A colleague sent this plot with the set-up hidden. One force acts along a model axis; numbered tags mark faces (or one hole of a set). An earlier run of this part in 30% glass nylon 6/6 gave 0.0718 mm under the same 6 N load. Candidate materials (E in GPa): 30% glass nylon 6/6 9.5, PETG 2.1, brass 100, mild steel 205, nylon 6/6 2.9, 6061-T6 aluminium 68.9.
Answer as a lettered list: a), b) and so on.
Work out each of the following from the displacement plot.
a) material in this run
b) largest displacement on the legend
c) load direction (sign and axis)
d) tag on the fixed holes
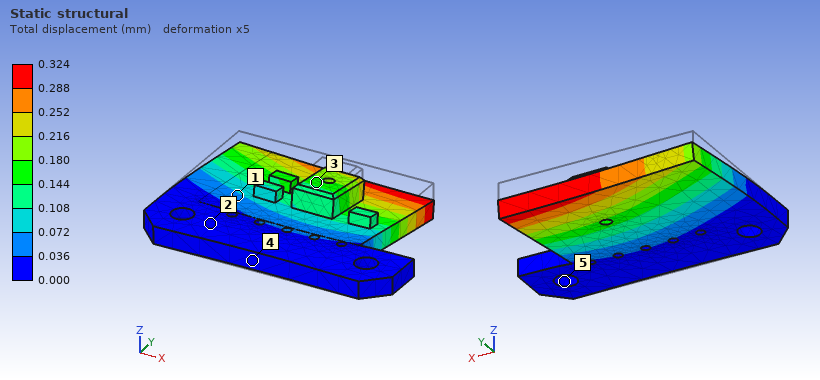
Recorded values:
a) PETG
b) 0.324 mm
c) -Z
d) 5
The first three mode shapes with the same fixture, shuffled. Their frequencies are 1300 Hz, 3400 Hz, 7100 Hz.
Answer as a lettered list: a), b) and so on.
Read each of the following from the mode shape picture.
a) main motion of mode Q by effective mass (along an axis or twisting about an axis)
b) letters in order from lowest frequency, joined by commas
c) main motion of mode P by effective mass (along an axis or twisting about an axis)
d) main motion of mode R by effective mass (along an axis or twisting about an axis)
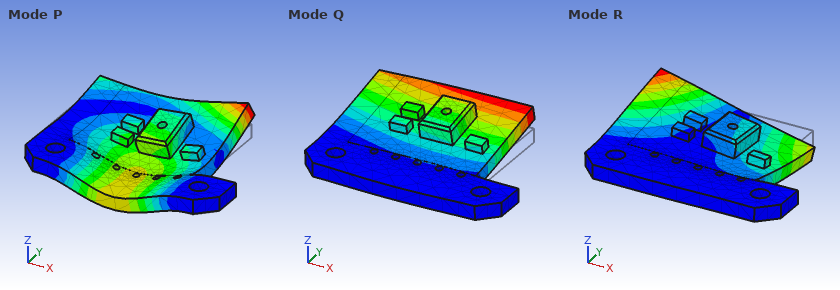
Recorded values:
a) along Z
b) Q, R, P
c) along Z
d) twisting about Y
